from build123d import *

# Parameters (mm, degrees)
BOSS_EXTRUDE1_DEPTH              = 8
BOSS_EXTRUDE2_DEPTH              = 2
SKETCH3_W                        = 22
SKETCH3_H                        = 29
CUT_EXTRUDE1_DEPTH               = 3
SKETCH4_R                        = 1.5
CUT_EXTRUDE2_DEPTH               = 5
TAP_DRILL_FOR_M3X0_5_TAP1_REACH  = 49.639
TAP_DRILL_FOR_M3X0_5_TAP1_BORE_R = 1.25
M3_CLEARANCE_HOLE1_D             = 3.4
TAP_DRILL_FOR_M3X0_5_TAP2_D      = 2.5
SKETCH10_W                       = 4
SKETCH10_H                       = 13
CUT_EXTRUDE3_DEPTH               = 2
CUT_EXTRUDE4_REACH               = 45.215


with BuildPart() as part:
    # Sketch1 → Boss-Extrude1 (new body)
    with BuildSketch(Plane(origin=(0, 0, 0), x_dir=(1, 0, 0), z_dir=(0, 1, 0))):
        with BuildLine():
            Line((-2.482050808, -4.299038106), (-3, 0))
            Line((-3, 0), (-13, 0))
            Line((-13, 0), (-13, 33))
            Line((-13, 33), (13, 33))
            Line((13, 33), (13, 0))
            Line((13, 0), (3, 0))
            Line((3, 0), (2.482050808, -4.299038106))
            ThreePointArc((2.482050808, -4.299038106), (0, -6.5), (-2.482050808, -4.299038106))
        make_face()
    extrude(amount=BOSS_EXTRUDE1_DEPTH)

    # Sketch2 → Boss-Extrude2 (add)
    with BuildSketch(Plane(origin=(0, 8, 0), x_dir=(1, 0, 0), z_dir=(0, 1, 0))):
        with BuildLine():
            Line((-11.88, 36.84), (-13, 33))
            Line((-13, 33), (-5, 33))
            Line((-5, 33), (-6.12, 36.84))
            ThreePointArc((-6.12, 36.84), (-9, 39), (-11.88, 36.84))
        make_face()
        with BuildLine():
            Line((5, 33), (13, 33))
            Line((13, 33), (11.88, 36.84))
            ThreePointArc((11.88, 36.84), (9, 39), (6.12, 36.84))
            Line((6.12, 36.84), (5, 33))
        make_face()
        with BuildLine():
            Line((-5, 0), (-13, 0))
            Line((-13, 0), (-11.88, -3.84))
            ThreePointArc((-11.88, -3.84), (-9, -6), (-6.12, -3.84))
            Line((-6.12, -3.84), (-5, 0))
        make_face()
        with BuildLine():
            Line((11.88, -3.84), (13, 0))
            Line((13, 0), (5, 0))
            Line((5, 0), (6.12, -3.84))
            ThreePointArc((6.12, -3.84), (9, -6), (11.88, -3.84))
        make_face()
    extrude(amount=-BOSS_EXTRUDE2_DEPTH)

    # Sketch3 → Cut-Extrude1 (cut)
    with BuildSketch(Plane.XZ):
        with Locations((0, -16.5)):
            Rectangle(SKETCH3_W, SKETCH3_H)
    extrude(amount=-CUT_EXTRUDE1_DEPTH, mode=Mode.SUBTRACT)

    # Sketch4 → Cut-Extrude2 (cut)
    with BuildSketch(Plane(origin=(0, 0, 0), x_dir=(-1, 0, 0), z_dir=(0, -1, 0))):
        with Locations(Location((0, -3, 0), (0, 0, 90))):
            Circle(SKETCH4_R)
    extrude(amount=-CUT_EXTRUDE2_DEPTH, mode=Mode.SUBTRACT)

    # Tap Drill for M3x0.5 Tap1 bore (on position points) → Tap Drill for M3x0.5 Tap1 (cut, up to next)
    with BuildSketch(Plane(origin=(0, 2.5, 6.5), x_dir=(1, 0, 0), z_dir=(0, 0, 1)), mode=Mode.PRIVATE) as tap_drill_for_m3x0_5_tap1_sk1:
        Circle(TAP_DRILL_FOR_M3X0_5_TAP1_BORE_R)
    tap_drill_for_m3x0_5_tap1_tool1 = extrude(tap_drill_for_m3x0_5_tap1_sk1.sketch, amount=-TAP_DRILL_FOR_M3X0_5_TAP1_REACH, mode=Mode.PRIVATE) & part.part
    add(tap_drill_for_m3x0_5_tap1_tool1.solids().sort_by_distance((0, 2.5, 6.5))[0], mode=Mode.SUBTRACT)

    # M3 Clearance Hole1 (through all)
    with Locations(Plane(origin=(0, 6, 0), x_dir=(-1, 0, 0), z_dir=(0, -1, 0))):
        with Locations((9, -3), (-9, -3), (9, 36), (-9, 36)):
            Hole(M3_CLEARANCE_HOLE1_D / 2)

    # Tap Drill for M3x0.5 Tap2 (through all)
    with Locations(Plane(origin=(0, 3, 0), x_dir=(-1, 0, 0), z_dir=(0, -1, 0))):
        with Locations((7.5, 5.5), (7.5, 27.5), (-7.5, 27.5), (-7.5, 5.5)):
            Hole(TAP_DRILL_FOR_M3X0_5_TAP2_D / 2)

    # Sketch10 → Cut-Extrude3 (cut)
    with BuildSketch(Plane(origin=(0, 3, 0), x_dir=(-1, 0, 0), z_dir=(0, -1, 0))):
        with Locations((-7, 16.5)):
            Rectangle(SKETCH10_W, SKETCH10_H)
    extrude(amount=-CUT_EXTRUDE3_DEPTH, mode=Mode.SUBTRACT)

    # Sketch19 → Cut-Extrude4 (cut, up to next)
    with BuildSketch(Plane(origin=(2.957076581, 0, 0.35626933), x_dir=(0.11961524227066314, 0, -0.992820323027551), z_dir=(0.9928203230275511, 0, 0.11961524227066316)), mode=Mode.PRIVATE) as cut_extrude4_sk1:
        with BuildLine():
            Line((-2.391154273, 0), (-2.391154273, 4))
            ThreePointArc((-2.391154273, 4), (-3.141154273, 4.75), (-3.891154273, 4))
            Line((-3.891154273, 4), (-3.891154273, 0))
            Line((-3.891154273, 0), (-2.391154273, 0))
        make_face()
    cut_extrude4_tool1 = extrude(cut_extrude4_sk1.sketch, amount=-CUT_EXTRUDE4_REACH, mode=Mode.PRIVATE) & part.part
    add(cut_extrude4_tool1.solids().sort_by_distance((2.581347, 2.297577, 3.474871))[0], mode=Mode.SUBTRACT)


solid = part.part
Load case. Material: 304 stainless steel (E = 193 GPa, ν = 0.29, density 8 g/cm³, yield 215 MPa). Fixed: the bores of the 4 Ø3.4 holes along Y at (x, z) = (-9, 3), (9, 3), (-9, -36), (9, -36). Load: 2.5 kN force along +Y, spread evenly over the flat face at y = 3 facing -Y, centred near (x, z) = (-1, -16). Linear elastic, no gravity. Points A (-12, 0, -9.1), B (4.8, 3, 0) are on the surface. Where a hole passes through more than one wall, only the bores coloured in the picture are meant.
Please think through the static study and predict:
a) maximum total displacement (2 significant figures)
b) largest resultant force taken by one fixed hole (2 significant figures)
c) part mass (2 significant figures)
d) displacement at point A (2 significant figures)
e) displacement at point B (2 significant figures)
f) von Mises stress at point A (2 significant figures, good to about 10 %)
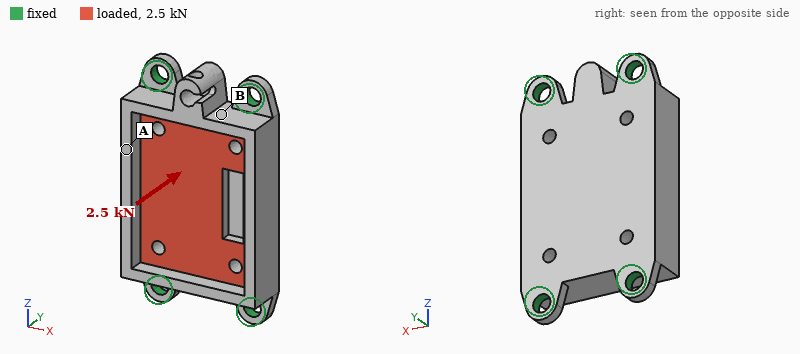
17 µm
1.0 kN
41 g
13 µm
5.0 µm
80 MPa
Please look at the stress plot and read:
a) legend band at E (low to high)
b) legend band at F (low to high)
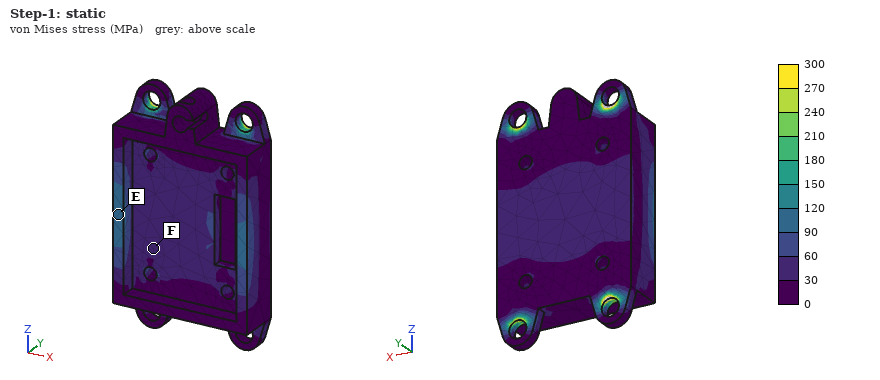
90 to 120 MPa
30 to 60 MPa
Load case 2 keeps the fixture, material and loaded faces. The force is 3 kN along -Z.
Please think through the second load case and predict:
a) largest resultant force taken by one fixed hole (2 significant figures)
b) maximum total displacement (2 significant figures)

820 N
3.2 µm
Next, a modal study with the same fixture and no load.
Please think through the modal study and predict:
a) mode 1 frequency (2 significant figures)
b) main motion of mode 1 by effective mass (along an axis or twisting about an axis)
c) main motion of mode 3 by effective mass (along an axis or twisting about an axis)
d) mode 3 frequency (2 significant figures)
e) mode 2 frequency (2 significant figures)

12 kHz
along Y
along X
22 kHz
16 kHz
